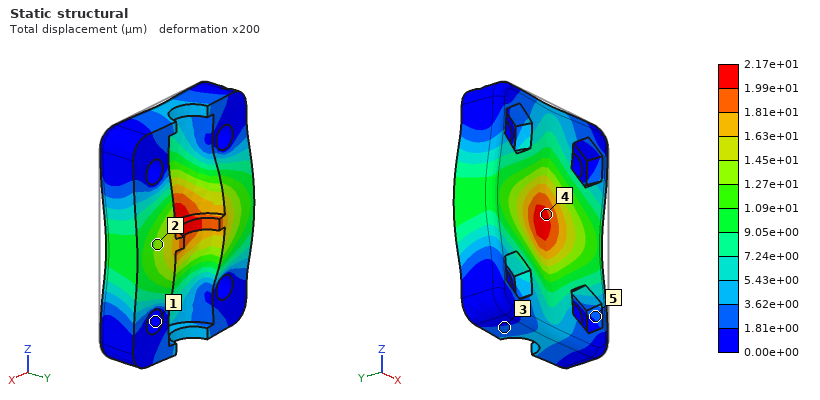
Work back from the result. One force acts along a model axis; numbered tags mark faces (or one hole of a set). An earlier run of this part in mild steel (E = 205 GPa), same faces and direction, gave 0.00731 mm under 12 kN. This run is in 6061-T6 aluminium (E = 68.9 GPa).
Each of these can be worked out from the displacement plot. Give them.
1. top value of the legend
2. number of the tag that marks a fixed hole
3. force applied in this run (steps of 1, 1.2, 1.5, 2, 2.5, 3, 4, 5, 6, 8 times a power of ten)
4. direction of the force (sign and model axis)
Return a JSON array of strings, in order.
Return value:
["2.17e+01 µm", "1", "12 kN", "+Y"]
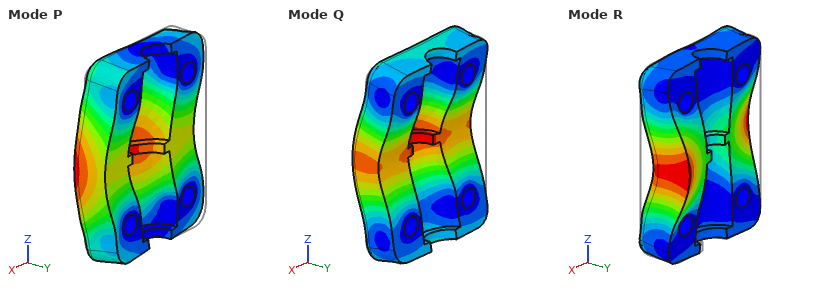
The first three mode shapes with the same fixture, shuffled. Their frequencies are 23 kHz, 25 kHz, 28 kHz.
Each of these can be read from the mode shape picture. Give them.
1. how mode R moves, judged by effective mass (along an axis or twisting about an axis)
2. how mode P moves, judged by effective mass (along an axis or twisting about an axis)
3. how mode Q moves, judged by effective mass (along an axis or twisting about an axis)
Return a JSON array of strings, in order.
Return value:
["twisting about Z", "along X", "along Y"]
